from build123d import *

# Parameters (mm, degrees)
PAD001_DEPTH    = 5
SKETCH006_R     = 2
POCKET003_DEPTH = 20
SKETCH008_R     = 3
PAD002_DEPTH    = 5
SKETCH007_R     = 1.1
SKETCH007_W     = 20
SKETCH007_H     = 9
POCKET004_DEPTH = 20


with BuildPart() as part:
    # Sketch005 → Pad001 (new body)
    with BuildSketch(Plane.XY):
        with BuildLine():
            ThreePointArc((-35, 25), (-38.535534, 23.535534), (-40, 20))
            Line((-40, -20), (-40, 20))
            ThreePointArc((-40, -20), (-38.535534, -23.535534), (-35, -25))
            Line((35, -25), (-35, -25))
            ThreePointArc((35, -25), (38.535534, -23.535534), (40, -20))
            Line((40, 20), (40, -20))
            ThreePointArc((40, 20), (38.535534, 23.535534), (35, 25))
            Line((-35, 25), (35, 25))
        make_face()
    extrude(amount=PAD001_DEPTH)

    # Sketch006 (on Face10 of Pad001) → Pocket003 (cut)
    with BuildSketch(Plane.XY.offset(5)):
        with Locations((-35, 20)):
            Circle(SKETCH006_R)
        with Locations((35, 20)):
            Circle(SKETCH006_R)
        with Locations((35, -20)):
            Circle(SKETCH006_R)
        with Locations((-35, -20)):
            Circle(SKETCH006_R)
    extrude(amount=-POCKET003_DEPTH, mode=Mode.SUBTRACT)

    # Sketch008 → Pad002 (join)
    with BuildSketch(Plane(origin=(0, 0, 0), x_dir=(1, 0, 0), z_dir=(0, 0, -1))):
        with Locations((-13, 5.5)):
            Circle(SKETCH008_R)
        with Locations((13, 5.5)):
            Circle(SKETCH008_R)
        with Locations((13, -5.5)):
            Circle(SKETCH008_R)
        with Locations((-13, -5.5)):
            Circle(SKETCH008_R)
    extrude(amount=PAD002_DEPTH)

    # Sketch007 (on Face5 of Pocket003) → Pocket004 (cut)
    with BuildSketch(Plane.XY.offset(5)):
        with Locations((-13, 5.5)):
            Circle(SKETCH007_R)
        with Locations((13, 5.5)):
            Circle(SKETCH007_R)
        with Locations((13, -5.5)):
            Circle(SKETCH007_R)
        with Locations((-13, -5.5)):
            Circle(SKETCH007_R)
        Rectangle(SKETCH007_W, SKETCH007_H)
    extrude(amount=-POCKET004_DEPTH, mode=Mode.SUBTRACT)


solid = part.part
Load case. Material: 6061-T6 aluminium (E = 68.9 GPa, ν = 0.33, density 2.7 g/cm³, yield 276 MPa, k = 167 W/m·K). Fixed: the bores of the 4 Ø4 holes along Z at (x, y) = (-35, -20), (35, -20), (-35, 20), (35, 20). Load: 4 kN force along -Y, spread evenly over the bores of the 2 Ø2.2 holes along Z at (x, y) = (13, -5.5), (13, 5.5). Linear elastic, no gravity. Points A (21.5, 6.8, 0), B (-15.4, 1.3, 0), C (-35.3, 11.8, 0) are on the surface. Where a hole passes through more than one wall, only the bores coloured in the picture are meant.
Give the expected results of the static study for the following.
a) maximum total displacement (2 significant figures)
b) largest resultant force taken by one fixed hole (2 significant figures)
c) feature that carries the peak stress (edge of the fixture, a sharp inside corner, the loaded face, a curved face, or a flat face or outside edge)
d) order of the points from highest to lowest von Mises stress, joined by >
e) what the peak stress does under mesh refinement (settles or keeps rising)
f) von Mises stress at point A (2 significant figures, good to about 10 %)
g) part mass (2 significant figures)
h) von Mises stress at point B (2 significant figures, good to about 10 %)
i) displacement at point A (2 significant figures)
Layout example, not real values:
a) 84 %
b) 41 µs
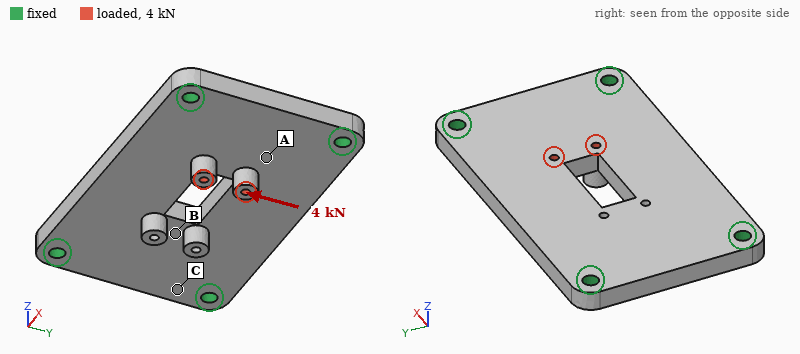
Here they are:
a) 44 µm
b) 1.9 kN
c) a sharp inside corner
d) A > B > C
e) keeps rising
f) 44 MPa
g) 52 g
h) 27 MPa
i) 13 µm
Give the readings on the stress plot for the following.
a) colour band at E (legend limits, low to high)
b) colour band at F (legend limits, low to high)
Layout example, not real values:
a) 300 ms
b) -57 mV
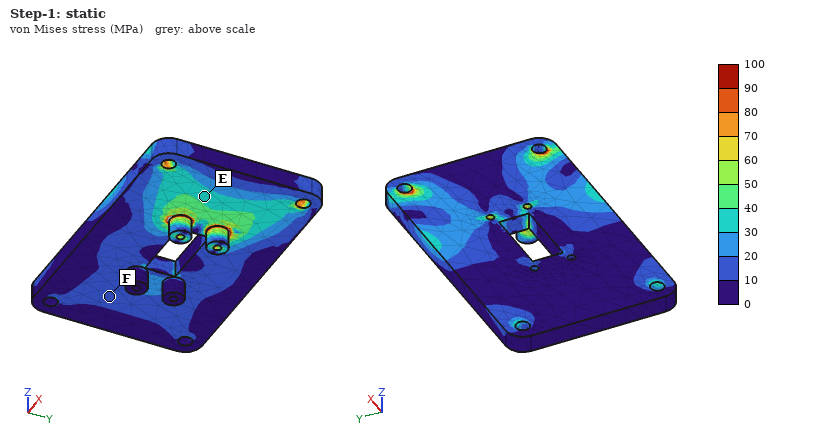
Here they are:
a) 30 to 40 MPa
b) 10 to 20 MPa
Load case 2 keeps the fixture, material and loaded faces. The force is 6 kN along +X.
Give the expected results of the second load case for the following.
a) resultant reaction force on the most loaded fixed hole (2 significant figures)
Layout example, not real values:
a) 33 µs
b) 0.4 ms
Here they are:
a) 2.1 kN
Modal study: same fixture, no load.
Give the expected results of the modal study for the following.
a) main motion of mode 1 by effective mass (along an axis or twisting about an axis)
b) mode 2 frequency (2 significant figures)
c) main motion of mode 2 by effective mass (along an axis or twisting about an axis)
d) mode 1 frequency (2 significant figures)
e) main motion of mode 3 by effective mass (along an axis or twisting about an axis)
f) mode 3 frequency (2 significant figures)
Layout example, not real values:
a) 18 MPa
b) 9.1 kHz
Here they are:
a) along Z
b) 6800 Hz
c) twisting about X
d) 4400 Hz
e) twisting about Y
f) 11 kHz
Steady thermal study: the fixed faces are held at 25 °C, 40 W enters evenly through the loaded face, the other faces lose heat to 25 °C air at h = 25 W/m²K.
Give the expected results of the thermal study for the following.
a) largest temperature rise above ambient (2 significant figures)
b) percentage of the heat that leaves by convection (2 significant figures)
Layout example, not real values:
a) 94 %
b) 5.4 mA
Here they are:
a) 32 K
b) 5.3 %
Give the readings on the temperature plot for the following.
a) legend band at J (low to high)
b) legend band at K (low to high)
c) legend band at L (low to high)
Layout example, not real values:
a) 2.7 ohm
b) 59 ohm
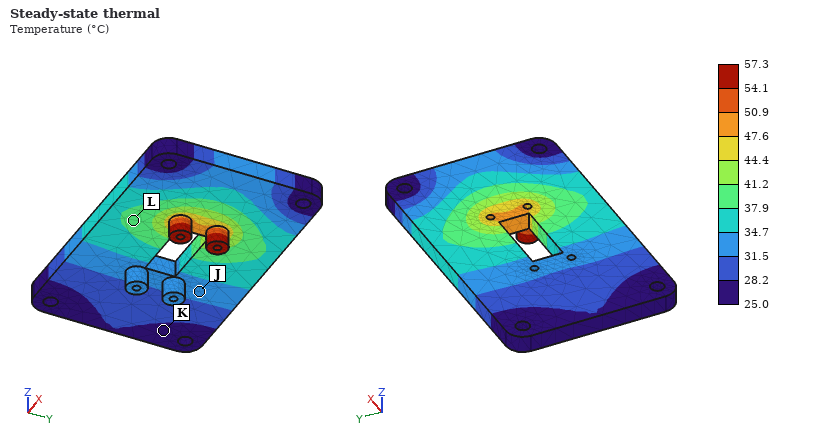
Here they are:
a) 31.5 to 34.7 °C
b) 25.0 to 28.2 °C
c) 37.9 to 41.2 °C
